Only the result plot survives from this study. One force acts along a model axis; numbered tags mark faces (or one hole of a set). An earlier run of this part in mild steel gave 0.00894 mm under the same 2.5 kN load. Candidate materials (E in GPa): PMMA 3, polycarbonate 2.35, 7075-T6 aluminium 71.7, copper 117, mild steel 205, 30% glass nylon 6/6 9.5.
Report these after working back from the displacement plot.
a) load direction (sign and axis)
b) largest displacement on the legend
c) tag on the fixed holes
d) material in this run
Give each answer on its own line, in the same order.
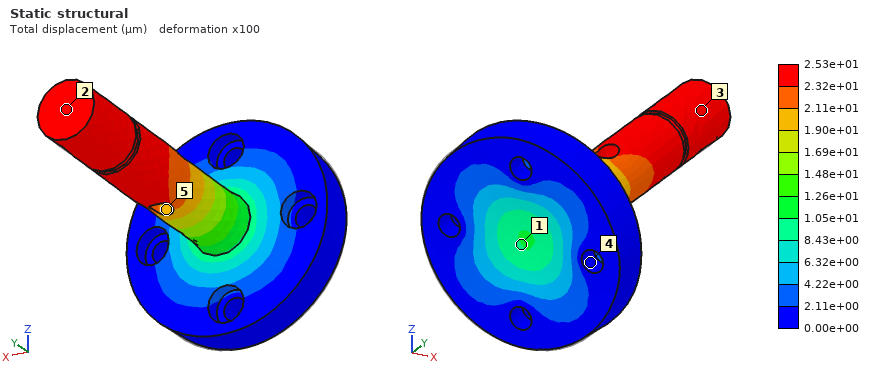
+Y
2.53e+01 µm
4
7075-T6 aluminium
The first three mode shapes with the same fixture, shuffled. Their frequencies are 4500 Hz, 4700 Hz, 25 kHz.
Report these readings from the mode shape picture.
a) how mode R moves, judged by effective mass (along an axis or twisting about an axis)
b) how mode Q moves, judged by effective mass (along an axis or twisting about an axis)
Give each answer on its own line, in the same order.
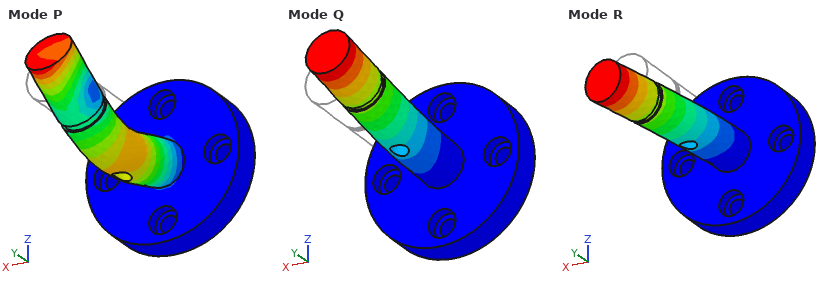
along X
along Z
